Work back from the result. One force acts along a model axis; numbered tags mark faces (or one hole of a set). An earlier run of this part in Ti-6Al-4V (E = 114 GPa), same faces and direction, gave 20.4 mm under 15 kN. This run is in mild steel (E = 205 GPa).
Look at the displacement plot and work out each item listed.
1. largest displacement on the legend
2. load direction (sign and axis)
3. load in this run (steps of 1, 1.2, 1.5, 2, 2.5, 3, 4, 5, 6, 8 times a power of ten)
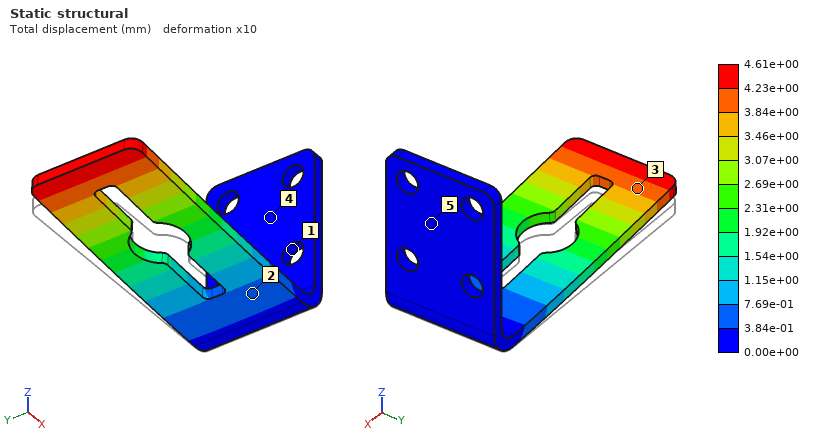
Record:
4.61e+00 mm
+Z
6 kN
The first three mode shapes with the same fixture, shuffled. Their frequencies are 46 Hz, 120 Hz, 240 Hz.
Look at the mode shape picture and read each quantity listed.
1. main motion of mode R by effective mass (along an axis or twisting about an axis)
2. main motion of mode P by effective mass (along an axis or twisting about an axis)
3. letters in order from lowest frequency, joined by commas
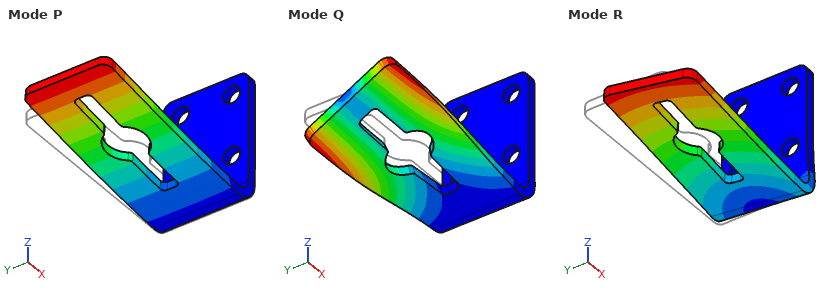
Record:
along Y
along Z
P, R, Q
